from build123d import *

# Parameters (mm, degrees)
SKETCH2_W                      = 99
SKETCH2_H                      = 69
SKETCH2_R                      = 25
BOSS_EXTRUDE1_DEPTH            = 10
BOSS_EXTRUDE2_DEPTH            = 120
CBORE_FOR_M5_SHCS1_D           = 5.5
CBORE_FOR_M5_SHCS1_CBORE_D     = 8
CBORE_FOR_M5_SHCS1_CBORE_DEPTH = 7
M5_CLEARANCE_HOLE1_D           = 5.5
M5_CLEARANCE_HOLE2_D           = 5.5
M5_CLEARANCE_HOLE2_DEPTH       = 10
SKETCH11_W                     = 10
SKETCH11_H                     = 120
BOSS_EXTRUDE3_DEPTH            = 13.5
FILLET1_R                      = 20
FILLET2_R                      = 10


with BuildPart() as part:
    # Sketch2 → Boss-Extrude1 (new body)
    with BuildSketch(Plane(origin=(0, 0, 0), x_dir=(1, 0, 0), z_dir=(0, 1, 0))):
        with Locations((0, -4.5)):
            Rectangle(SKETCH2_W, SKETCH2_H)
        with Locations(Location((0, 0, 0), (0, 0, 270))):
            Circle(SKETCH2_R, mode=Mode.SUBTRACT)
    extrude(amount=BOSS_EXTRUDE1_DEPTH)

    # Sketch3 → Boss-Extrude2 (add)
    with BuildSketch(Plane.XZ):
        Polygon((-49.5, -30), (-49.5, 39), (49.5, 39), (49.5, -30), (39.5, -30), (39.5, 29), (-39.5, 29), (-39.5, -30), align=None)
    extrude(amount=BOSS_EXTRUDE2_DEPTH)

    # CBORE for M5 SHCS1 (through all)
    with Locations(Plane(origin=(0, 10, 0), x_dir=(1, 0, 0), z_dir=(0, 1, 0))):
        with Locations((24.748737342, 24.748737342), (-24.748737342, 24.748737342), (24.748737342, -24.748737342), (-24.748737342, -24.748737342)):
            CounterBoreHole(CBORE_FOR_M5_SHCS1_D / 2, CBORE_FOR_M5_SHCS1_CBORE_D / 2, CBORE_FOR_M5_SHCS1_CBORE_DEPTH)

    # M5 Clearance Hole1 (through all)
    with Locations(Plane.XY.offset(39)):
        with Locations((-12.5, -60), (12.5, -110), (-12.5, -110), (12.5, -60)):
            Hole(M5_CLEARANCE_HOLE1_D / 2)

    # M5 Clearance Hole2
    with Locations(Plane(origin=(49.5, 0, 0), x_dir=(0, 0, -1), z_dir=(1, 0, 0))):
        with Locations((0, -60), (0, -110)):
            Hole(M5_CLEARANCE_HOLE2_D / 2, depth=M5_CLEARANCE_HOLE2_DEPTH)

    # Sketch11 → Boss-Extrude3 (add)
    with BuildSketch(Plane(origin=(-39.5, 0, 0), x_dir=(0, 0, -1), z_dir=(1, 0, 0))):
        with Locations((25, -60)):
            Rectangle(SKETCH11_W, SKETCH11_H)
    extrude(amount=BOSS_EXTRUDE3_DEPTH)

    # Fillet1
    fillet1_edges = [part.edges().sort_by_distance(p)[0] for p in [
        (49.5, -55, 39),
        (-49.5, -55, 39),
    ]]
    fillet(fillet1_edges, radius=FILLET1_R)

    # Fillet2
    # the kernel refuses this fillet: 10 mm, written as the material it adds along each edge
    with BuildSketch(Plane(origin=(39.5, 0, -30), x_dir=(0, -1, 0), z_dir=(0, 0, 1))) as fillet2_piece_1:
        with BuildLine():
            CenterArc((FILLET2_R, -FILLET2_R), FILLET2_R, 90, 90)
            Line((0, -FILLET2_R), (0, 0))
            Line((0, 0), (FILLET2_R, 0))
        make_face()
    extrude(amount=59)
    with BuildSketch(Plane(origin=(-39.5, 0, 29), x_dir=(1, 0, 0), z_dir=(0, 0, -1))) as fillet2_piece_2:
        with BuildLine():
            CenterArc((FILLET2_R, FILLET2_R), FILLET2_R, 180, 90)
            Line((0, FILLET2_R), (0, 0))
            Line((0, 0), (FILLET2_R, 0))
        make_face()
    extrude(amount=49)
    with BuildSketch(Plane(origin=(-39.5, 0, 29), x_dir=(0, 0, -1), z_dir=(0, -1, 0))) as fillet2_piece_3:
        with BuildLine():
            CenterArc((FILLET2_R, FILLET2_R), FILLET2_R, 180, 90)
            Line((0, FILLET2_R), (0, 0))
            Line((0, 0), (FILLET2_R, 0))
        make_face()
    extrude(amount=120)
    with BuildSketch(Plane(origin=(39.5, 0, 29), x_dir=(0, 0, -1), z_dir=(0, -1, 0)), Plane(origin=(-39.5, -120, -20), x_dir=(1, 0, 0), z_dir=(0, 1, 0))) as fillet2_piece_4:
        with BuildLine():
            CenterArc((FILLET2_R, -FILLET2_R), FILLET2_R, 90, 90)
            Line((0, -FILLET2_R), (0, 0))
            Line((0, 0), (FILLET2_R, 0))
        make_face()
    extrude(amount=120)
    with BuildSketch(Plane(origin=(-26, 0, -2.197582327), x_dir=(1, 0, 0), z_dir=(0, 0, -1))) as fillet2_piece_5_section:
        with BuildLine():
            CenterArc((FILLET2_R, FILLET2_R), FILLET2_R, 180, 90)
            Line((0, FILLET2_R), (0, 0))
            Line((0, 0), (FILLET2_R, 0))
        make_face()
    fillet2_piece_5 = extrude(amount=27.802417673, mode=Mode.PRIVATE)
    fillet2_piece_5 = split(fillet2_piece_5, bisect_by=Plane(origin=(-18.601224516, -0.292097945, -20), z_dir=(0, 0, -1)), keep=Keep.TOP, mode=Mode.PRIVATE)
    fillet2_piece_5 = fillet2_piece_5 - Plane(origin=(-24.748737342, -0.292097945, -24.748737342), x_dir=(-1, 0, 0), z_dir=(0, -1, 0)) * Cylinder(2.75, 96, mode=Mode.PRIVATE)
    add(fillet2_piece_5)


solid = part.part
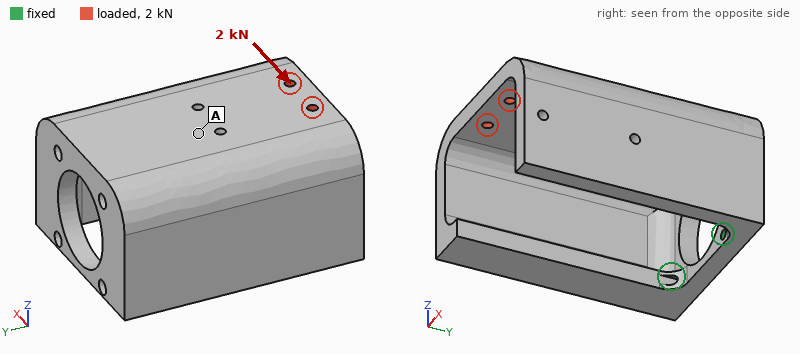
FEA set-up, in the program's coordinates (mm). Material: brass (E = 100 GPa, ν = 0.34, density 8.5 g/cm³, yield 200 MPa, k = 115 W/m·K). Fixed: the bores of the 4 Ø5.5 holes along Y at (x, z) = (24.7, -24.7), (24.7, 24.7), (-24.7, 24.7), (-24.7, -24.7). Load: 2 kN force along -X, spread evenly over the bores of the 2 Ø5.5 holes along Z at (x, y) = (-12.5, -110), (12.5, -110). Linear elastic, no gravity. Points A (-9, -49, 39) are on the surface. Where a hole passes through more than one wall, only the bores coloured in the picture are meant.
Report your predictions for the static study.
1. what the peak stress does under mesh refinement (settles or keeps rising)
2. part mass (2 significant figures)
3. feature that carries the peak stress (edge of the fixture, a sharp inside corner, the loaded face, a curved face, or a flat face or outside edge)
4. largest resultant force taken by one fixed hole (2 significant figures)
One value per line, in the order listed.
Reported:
keeps rising
2.6 kg
edge of the fixture
4.1 kN
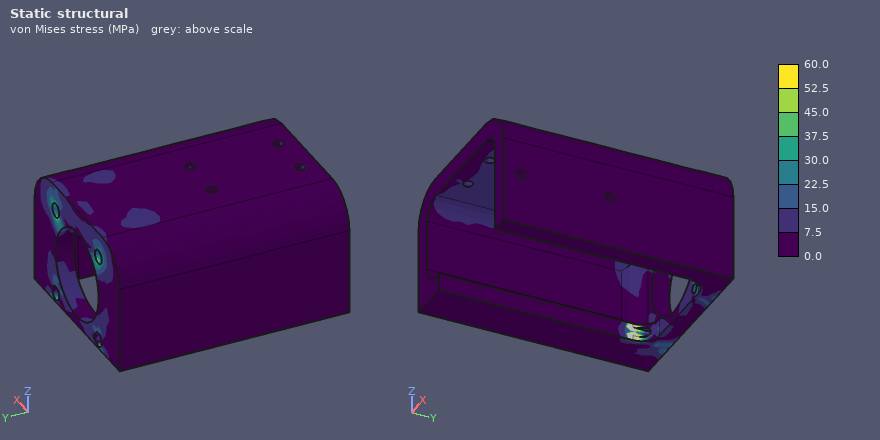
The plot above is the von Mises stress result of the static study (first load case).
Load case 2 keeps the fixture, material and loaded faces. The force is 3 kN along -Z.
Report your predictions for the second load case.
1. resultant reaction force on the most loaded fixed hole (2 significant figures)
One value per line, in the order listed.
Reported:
3.8 kN
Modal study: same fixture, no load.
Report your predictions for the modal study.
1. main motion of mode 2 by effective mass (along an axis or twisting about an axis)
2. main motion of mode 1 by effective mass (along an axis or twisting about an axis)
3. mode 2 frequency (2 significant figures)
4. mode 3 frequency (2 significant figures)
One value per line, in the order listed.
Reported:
along Z
along X
800 Hz
1200 Hz
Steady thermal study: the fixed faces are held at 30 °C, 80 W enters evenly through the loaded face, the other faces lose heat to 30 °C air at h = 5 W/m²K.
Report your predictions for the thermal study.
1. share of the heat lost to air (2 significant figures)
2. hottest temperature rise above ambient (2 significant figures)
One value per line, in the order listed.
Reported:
10 %
69 K
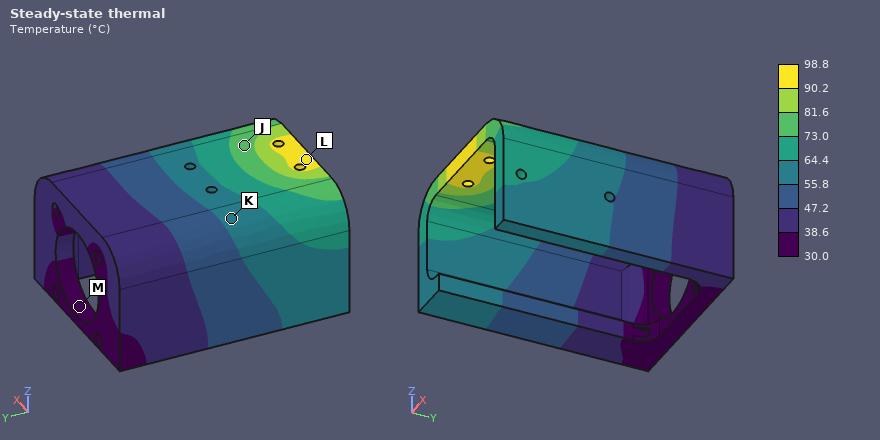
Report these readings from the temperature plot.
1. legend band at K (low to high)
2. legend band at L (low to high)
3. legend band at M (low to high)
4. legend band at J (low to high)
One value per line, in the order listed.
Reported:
55.8 to 64.4 °C
90.2 to 98.8 °C
30.0 to 38.6 °C
73.0 to 81.6 °C
